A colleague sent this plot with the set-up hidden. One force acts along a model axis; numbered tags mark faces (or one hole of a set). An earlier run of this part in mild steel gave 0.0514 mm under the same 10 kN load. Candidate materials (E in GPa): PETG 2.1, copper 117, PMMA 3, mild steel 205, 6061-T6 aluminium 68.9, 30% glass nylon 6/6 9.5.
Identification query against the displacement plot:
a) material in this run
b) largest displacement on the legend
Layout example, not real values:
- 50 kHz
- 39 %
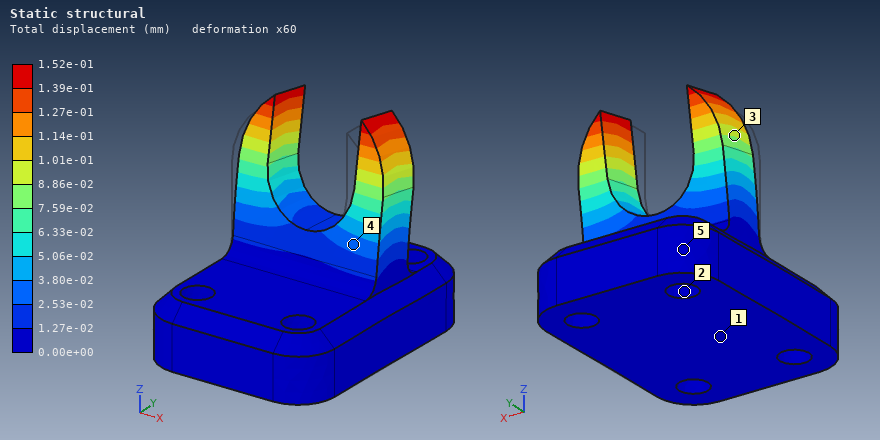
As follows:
- 6061-T6 aluminium
- 1.52e-01 mm
